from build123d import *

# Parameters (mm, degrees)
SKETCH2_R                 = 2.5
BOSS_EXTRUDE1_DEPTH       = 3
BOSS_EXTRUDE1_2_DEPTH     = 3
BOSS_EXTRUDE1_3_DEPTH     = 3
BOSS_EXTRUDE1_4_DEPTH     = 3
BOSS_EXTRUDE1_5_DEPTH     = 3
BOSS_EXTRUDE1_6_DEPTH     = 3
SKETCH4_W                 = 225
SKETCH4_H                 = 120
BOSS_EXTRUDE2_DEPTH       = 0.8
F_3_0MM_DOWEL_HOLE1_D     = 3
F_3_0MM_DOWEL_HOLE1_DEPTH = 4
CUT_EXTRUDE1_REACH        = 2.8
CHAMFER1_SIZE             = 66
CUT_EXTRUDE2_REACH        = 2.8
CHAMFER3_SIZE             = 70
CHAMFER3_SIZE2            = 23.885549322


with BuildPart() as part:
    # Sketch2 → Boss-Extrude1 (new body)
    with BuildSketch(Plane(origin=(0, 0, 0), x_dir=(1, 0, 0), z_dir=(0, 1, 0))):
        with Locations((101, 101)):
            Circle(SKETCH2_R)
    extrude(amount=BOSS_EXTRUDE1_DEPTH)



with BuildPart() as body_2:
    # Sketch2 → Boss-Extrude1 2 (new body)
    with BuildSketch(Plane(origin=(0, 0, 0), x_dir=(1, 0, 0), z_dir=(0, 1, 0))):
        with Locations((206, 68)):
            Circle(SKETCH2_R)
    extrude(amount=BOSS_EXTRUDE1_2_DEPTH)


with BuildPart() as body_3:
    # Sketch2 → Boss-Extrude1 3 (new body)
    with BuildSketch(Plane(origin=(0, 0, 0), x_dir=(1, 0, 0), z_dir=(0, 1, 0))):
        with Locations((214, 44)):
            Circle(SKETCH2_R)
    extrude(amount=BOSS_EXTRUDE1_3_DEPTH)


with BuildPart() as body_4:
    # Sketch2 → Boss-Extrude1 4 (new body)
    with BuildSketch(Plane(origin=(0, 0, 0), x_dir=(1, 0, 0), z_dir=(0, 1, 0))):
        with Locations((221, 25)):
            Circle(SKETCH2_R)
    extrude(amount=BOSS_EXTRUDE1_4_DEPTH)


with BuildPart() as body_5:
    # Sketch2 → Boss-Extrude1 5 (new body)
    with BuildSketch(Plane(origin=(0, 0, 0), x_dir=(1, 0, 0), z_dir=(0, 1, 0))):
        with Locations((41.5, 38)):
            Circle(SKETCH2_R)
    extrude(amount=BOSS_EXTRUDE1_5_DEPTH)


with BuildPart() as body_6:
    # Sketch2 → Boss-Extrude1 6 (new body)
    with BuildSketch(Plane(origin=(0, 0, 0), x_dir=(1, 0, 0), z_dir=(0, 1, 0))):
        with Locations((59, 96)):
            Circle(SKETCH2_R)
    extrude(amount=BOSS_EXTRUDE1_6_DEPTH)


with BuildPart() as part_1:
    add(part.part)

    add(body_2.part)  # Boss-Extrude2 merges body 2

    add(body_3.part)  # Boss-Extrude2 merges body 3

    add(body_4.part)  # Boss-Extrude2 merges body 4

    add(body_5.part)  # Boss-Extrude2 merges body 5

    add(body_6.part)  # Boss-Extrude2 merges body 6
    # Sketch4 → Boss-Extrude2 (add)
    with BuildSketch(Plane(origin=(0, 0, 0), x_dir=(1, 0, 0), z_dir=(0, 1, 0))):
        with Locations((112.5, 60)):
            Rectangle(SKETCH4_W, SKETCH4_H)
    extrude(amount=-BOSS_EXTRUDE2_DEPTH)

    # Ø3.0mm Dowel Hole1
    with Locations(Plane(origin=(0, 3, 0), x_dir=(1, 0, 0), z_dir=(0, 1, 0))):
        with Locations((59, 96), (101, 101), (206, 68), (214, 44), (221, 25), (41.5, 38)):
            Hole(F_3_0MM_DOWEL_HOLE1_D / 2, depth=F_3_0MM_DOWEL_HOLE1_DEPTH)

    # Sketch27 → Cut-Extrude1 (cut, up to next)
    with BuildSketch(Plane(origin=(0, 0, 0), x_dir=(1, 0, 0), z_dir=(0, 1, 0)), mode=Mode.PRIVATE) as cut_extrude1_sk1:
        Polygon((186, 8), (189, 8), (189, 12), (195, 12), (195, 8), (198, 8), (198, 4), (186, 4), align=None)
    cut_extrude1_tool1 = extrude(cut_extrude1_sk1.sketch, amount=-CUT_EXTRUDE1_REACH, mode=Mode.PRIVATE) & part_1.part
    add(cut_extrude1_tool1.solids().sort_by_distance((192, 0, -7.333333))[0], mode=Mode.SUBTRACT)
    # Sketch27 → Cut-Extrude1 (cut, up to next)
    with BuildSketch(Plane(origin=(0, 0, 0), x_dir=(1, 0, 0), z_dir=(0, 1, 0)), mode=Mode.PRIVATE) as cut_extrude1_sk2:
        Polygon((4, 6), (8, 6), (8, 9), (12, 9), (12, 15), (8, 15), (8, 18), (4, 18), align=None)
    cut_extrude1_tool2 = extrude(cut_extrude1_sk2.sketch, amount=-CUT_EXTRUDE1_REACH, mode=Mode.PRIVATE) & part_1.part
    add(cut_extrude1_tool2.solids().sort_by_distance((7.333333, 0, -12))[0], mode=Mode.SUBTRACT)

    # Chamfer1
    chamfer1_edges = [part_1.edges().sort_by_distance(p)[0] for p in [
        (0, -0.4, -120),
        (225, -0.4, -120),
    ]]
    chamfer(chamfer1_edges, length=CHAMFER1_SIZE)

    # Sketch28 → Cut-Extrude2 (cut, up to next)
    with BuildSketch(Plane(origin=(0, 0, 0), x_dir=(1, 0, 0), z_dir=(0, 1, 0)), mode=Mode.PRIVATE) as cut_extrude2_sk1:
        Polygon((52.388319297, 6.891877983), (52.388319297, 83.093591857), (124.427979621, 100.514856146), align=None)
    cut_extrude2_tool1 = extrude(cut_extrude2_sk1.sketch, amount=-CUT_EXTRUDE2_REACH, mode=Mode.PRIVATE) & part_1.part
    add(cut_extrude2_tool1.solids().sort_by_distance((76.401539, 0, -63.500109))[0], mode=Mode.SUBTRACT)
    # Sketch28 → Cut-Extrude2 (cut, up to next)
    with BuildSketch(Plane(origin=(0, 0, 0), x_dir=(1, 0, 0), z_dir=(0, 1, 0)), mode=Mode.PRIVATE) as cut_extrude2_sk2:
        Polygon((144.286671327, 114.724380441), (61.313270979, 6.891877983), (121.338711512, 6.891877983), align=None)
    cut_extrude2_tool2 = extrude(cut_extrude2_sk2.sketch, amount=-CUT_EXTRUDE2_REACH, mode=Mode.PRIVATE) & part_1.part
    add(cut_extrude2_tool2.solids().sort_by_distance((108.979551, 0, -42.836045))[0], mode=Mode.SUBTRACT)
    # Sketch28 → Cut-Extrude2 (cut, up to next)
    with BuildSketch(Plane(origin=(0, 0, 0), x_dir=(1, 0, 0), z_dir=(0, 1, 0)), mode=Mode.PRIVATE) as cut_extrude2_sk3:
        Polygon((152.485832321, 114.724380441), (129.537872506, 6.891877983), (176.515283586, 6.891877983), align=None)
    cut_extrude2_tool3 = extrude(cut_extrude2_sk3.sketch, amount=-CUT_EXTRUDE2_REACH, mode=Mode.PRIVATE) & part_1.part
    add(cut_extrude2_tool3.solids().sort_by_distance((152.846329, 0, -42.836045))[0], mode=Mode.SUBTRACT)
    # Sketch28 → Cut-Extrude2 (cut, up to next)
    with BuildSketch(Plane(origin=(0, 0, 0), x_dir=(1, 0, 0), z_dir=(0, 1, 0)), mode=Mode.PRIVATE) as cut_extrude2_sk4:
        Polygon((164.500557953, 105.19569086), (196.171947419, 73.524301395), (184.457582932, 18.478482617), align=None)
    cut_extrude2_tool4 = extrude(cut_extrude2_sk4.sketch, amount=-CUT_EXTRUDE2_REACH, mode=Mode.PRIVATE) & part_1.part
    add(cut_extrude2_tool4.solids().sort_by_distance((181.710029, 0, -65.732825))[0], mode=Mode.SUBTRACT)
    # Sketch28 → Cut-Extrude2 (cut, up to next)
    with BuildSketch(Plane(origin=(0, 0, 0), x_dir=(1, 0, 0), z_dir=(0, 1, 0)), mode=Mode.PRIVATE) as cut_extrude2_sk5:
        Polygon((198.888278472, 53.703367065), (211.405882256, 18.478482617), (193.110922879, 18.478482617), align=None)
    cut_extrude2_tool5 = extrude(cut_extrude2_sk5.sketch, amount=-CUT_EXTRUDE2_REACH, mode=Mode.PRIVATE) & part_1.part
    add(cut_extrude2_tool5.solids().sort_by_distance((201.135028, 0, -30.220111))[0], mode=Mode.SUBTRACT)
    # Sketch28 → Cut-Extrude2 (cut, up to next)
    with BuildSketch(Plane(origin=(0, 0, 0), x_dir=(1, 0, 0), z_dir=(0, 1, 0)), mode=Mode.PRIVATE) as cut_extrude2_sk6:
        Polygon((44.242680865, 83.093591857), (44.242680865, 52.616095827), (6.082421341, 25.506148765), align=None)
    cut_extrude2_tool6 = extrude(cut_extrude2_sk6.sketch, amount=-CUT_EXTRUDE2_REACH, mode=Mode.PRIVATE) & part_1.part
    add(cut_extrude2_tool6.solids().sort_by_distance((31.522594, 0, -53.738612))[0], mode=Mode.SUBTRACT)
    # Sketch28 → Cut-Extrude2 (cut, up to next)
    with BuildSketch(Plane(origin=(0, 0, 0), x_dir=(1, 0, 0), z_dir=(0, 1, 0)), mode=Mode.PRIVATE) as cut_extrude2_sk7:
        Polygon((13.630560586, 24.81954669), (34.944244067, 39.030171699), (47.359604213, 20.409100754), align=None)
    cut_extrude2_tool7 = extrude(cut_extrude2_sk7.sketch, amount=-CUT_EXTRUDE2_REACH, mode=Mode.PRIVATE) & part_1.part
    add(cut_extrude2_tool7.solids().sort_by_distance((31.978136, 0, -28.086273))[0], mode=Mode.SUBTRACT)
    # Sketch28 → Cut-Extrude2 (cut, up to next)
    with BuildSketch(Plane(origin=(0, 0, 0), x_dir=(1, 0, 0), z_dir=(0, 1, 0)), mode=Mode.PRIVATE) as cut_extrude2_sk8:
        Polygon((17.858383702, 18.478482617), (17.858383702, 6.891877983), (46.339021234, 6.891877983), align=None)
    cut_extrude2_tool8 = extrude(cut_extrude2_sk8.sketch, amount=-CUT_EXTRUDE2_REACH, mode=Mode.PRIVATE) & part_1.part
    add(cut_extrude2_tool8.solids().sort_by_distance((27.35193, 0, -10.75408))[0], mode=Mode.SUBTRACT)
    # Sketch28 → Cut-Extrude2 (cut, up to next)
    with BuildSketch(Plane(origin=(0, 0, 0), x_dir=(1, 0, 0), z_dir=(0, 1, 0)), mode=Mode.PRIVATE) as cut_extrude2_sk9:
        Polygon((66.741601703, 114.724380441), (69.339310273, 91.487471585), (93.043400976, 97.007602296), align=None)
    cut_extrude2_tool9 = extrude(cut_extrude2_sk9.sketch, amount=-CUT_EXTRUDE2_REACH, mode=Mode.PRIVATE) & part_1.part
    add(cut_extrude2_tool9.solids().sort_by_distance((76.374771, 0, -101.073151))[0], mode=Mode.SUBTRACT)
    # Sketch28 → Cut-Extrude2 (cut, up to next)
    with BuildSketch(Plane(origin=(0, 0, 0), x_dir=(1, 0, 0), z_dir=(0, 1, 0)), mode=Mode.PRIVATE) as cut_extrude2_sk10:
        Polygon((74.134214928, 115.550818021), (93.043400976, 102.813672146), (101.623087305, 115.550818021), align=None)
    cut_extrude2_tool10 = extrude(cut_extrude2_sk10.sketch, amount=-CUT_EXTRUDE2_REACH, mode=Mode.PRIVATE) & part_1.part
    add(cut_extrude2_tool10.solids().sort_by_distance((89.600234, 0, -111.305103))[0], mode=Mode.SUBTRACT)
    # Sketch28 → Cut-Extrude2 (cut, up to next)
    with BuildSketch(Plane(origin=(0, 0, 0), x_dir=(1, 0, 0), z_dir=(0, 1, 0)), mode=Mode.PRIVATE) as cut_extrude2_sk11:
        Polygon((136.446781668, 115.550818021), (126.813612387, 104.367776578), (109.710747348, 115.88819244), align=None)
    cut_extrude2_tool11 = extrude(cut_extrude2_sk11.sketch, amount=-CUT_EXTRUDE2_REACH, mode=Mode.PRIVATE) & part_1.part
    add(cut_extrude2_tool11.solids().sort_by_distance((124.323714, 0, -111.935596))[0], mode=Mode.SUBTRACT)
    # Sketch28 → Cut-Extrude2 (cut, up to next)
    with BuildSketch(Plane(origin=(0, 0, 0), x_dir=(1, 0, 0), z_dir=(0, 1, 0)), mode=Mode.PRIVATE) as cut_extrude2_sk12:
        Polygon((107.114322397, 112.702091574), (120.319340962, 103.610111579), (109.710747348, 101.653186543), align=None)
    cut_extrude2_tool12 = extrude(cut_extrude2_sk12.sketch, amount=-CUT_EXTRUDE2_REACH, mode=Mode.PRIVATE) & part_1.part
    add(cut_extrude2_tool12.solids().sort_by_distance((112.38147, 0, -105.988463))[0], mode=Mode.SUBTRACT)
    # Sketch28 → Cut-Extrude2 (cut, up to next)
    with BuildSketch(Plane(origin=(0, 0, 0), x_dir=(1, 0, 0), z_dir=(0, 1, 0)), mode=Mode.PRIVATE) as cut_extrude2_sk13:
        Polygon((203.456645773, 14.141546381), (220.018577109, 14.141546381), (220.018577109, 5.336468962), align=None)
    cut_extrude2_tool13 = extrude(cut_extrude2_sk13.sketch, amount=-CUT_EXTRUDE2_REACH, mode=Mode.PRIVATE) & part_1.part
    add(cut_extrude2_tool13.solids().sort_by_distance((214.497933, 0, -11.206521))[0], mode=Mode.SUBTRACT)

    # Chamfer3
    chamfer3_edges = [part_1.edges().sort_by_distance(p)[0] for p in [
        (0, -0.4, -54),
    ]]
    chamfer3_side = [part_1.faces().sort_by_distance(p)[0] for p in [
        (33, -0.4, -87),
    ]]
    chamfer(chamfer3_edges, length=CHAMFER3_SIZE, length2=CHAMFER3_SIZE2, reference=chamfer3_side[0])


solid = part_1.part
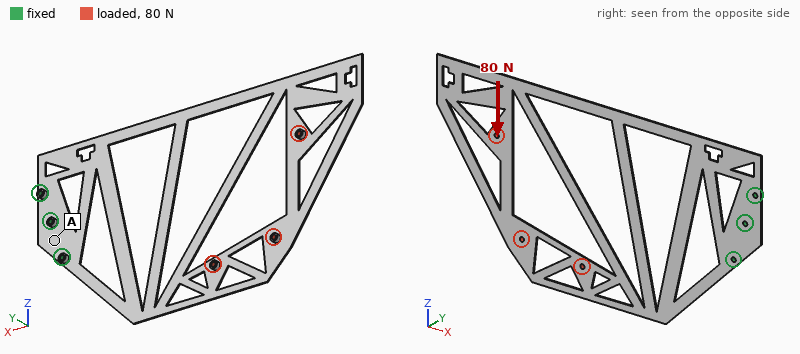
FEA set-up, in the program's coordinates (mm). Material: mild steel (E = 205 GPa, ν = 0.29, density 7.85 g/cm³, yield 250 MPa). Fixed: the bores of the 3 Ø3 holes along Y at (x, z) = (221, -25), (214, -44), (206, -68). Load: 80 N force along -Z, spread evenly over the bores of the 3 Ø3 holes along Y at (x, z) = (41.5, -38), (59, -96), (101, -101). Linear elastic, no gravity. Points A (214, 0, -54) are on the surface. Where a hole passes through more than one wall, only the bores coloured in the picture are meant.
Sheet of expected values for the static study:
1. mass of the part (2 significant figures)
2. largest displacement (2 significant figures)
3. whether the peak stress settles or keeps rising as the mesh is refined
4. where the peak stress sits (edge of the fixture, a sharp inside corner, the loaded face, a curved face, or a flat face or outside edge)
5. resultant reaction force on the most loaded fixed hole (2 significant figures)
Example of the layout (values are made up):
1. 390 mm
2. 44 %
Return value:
1. 66 g
2. 2.7 mm
3. keeps rising
4. a sharp inside corner
5. 250 N
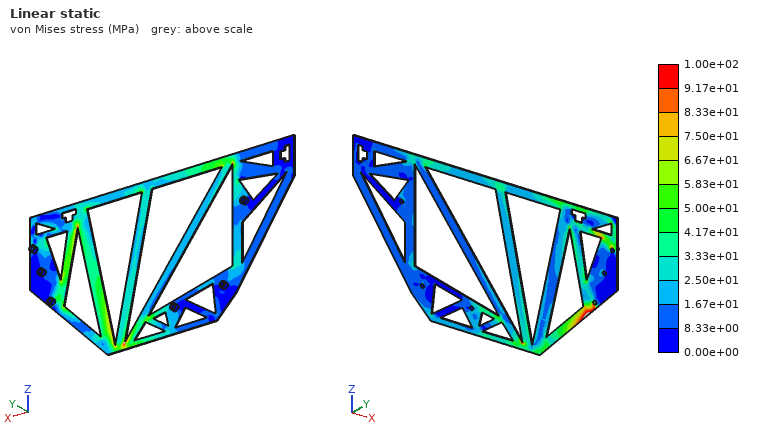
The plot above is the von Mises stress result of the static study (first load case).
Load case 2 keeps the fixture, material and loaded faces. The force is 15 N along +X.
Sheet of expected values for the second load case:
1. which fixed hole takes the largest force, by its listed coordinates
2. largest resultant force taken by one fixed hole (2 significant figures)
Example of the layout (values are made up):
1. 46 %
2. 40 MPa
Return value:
1. (206, -68)
2. 20 N
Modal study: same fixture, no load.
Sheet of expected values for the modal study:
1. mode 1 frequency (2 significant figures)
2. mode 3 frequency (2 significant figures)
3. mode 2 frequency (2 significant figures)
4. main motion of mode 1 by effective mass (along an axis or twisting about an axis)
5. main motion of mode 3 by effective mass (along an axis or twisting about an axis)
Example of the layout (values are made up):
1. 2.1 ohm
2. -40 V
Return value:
1. 9.9 Hz
2. 70 Hz
3. 40 Hz
4. along Y
5. along Y
